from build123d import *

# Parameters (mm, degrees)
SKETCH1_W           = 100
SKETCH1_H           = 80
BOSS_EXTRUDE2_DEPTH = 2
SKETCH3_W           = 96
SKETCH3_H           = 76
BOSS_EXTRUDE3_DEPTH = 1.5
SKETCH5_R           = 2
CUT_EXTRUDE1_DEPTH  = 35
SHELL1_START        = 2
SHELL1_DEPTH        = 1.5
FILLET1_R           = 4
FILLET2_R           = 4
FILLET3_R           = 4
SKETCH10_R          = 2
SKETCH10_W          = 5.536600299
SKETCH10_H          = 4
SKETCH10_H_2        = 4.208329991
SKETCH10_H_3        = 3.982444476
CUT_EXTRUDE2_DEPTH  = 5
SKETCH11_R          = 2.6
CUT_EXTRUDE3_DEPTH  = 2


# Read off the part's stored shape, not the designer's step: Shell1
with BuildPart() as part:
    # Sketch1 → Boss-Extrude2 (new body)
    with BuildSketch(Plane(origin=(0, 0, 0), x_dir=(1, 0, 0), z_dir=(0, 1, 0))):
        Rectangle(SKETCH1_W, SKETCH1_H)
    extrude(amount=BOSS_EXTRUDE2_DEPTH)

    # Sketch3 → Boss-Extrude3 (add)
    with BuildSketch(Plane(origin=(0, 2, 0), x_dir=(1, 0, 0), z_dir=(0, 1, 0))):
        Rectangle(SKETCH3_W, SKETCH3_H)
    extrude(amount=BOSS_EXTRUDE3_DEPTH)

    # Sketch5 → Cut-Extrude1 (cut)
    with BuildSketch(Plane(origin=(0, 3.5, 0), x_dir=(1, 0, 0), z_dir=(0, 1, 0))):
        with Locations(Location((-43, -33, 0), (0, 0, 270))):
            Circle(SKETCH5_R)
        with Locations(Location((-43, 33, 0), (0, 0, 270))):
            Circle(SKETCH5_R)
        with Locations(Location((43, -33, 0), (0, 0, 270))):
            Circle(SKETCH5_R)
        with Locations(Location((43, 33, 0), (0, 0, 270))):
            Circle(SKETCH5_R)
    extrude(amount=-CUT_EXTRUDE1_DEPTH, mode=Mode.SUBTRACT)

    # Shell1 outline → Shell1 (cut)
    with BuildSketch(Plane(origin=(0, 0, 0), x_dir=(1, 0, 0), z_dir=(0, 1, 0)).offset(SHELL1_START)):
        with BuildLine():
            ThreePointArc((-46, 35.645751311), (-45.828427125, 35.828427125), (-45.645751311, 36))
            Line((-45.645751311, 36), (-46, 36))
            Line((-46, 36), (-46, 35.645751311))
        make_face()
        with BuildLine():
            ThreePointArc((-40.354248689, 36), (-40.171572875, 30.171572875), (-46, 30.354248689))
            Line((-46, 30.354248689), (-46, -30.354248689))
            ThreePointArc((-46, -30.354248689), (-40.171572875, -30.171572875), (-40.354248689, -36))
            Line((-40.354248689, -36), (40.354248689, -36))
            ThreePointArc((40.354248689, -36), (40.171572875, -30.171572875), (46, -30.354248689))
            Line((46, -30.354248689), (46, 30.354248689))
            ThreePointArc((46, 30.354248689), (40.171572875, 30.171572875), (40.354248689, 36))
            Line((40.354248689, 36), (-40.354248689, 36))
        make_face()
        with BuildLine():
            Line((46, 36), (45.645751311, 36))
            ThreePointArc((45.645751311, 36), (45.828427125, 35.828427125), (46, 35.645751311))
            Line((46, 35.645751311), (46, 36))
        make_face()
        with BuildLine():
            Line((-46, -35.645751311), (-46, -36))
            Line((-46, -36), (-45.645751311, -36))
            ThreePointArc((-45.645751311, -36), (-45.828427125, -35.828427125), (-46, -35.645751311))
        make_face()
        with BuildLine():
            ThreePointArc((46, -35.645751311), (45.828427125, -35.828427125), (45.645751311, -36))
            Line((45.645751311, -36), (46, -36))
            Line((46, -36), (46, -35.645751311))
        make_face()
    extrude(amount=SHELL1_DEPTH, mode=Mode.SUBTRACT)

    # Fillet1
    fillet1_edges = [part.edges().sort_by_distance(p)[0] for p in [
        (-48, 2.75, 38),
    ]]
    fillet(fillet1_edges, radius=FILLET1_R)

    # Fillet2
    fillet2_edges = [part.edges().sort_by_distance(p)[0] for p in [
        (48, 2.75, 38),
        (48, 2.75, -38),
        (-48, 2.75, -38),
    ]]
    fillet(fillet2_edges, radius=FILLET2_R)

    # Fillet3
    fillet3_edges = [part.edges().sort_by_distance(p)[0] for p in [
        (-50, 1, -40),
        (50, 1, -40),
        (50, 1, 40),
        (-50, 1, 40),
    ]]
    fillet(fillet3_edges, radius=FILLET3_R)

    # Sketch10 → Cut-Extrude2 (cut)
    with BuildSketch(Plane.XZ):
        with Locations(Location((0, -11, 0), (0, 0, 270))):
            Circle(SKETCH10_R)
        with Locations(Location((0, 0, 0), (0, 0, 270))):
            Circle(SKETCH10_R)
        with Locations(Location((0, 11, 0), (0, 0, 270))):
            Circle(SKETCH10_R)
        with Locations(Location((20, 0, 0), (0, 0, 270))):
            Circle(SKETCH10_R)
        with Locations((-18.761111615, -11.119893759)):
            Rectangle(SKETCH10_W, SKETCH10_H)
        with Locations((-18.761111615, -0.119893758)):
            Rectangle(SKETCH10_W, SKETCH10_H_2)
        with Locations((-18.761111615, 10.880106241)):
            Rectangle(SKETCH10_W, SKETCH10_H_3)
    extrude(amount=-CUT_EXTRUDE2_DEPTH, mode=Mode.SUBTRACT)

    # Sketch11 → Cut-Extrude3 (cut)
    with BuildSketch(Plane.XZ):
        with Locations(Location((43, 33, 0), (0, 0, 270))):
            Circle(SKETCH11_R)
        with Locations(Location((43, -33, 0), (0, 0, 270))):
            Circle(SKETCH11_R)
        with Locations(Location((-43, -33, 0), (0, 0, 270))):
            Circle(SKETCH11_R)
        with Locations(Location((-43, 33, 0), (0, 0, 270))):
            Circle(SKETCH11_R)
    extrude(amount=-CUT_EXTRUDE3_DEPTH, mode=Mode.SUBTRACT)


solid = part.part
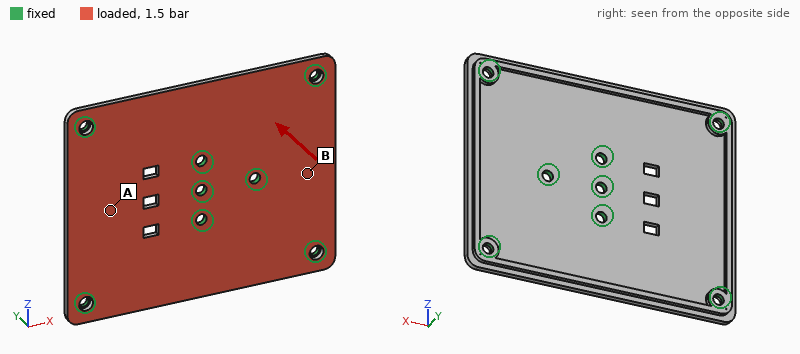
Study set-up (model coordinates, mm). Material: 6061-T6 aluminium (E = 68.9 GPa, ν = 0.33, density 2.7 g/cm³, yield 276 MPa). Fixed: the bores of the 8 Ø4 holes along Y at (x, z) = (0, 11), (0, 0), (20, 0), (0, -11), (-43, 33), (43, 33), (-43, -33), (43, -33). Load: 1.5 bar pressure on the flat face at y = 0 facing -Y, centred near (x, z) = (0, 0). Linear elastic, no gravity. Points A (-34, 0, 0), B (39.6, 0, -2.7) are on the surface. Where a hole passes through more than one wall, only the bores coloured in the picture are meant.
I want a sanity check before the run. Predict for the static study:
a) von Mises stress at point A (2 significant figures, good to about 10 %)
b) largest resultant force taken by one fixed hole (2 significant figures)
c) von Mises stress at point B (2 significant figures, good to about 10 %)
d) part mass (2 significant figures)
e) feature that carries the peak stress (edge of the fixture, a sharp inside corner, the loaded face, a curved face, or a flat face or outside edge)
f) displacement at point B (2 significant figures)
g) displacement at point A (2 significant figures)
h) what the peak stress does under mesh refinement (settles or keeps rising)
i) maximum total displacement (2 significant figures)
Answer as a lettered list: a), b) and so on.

a) 20 MPa
b) 280 N
c) 9.6 MPa
d) 45 g
e) edge of the fixture
f) 0.036 mm
g) 0.082 mm
h) keeps rising
i) 0.11 mm
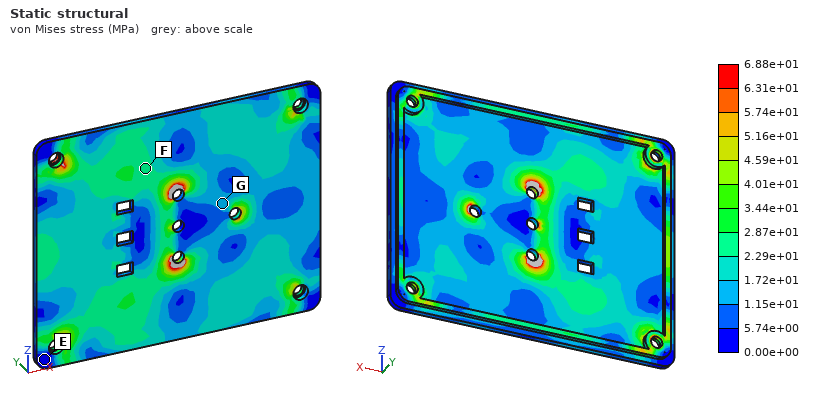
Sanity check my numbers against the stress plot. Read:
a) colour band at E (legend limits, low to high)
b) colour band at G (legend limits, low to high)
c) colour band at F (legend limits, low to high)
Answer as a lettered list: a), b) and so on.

a) 0.00e+00 to 5.74e+00 MPa
b) 1.15e+01 to 1.72e+01 MPa
c) 2.29e+01 to 2.87e+01 MPa
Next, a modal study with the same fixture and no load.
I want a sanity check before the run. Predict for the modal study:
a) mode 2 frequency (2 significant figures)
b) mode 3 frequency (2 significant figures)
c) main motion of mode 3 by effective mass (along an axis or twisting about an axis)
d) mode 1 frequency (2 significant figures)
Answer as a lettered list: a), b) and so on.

a) 3000 Hz
b) 3200 Hz
c) along Y
d) 2900 Hz
